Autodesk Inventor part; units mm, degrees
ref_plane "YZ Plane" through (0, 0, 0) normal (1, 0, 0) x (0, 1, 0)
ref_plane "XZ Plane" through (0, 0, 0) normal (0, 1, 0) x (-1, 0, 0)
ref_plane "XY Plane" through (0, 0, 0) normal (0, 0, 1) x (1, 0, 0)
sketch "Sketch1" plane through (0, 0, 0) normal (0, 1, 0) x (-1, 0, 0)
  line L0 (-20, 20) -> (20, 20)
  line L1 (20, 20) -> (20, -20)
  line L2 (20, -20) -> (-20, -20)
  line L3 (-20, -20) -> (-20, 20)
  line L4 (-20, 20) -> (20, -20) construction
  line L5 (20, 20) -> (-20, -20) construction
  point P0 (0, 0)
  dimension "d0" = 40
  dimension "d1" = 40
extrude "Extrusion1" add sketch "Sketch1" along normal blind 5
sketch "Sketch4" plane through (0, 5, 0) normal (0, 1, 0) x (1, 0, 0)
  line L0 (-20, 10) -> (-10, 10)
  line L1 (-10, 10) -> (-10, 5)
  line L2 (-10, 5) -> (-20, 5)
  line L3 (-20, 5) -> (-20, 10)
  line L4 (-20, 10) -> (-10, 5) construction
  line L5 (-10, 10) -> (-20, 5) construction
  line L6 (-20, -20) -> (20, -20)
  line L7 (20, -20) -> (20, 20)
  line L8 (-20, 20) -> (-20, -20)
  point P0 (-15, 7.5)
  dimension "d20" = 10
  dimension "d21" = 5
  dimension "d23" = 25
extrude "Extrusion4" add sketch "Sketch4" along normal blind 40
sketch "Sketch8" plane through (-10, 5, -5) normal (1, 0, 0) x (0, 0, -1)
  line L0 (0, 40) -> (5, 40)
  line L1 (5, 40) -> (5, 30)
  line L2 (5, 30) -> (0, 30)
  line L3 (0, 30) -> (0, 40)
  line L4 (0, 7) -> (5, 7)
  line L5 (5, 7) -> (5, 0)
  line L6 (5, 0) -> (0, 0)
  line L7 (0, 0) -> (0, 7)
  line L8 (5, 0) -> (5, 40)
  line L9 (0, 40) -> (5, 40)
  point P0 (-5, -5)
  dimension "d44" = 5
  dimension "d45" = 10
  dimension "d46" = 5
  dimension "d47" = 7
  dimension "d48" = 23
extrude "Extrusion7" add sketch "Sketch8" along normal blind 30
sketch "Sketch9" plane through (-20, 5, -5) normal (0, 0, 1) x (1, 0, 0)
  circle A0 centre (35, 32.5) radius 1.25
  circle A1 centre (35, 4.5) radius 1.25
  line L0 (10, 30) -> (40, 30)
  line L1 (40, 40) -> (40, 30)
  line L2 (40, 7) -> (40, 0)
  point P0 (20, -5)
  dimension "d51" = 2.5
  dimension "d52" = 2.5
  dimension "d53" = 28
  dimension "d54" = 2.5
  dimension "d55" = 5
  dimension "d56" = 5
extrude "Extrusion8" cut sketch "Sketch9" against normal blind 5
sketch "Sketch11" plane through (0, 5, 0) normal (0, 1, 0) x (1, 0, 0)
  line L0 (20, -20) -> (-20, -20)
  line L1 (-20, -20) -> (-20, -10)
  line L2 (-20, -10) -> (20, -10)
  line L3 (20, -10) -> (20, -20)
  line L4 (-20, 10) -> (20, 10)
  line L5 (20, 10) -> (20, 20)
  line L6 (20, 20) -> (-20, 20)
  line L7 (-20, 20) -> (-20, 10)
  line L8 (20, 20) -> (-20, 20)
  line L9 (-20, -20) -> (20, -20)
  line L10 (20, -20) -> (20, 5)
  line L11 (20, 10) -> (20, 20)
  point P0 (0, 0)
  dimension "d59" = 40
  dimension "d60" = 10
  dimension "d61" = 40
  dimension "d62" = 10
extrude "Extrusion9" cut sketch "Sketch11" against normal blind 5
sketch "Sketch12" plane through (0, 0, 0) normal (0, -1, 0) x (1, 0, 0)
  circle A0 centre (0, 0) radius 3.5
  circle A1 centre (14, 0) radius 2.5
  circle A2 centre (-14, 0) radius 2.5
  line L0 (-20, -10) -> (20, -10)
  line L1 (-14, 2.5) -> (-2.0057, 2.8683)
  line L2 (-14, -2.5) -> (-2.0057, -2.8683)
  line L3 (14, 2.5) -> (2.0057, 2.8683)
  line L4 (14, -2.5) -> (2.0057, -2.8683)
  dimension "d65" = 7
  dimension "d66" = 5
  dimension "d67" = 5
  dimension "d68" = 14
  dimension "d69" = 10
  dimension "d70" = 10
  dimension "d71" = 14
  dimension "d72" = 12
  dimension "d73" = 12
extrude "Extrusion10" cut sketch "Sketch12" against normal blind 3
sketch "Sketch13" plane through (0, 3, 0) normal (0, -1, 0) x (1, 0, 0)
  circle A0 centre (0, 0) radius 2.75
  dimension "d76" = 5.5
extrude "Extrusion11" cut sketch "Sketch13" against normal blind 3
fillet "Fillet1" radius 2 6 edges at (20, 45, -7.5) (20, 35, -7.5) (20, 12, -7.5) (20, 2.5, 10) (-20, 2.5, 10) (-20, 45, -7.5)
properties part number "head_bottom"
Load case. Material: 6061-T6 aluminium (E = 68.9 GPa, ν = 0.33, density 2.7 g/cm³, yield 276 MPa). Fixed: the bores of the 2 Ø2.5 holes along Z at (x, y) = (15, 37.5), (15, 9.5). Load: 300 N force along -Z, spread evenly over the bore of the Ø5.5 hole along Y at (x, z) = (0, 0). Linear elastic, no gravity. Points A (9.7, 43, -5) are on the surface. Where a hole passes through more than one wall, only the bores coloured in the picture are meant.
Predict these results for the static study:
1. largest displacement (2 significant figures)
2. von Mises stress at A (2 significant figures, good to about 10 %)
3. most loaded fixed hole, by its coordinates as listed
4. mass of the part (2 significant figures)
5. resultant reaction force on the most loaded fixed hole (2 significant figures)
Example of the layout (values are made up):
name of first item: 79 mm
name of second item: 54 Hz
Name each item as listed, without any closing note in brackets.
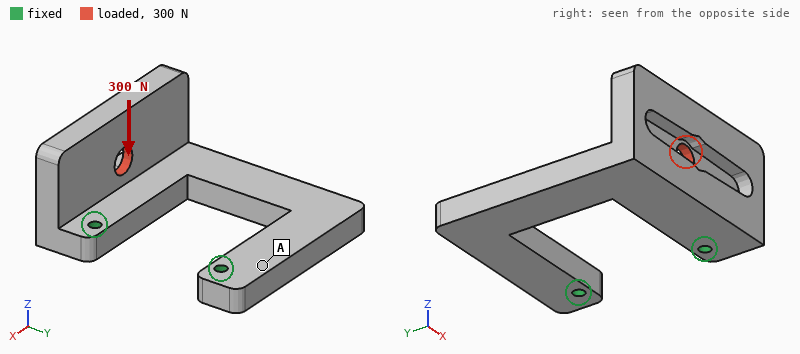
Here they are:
largest displacement: 0.10 mm
von Mises stress at A: 10 MPa
most loaded fixed hole, by its coordinates as listed: (15, 9.5)
mass of the part: 21 g
resultant reaction force on the most loaded fixed hole: 290 N
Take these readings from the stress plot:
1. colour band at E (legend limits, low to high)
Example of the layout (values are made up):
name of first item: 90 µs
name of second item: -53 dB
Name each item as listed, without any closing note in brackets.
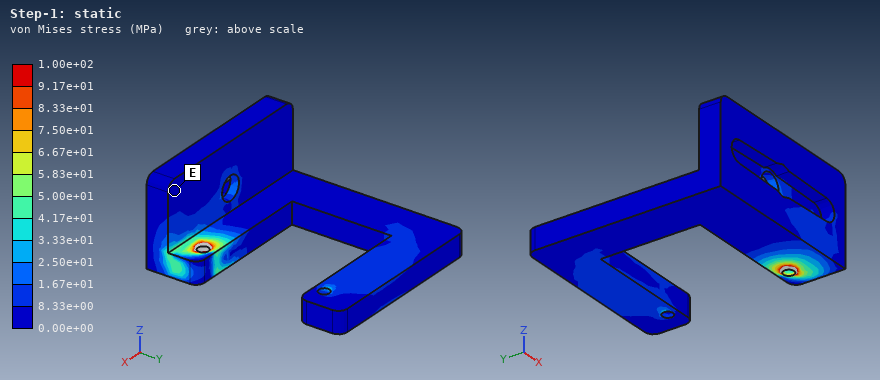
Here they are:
colour band at E: 0.00e+00 to 8.33e+00 MPa
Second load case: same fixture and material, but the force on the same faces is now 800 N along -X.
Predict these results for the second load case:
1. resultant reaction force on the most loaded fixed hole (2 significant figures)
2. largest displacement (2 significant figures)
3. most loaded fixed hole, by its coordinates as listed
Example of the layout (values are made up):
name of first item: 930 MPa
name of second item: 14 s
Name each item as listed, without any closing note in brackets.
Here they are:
resultant reaction force on the most loaded fixed hole: 850 N
largest displacement: 0.14 mm
most loaded fixed hole, by its coordinates as listed: (15, 9.5)
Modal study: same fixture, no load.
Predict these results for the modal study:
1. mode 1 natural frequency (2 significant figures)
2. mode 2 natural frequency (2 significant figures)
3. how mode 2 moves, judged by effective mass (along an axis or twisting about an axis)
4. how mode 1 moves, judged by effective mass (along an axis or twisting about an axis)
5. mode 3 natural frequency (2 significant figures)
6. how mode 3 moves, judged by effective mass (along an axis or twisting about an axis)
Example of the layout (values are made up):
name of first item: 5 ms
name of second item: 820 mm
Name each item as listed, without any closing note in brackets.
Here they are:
mode 1 natural frequency: 2400 Hz
mode 2 natural frequency: 3600 Hz
how mode 2 moves, judged by effective mass: along Y
how mode 1 moves, judged by effective mass: along Z
mode 3 natural frequency: 4500 Hz
how mode 3 moves, judged by effective mass: along Y
